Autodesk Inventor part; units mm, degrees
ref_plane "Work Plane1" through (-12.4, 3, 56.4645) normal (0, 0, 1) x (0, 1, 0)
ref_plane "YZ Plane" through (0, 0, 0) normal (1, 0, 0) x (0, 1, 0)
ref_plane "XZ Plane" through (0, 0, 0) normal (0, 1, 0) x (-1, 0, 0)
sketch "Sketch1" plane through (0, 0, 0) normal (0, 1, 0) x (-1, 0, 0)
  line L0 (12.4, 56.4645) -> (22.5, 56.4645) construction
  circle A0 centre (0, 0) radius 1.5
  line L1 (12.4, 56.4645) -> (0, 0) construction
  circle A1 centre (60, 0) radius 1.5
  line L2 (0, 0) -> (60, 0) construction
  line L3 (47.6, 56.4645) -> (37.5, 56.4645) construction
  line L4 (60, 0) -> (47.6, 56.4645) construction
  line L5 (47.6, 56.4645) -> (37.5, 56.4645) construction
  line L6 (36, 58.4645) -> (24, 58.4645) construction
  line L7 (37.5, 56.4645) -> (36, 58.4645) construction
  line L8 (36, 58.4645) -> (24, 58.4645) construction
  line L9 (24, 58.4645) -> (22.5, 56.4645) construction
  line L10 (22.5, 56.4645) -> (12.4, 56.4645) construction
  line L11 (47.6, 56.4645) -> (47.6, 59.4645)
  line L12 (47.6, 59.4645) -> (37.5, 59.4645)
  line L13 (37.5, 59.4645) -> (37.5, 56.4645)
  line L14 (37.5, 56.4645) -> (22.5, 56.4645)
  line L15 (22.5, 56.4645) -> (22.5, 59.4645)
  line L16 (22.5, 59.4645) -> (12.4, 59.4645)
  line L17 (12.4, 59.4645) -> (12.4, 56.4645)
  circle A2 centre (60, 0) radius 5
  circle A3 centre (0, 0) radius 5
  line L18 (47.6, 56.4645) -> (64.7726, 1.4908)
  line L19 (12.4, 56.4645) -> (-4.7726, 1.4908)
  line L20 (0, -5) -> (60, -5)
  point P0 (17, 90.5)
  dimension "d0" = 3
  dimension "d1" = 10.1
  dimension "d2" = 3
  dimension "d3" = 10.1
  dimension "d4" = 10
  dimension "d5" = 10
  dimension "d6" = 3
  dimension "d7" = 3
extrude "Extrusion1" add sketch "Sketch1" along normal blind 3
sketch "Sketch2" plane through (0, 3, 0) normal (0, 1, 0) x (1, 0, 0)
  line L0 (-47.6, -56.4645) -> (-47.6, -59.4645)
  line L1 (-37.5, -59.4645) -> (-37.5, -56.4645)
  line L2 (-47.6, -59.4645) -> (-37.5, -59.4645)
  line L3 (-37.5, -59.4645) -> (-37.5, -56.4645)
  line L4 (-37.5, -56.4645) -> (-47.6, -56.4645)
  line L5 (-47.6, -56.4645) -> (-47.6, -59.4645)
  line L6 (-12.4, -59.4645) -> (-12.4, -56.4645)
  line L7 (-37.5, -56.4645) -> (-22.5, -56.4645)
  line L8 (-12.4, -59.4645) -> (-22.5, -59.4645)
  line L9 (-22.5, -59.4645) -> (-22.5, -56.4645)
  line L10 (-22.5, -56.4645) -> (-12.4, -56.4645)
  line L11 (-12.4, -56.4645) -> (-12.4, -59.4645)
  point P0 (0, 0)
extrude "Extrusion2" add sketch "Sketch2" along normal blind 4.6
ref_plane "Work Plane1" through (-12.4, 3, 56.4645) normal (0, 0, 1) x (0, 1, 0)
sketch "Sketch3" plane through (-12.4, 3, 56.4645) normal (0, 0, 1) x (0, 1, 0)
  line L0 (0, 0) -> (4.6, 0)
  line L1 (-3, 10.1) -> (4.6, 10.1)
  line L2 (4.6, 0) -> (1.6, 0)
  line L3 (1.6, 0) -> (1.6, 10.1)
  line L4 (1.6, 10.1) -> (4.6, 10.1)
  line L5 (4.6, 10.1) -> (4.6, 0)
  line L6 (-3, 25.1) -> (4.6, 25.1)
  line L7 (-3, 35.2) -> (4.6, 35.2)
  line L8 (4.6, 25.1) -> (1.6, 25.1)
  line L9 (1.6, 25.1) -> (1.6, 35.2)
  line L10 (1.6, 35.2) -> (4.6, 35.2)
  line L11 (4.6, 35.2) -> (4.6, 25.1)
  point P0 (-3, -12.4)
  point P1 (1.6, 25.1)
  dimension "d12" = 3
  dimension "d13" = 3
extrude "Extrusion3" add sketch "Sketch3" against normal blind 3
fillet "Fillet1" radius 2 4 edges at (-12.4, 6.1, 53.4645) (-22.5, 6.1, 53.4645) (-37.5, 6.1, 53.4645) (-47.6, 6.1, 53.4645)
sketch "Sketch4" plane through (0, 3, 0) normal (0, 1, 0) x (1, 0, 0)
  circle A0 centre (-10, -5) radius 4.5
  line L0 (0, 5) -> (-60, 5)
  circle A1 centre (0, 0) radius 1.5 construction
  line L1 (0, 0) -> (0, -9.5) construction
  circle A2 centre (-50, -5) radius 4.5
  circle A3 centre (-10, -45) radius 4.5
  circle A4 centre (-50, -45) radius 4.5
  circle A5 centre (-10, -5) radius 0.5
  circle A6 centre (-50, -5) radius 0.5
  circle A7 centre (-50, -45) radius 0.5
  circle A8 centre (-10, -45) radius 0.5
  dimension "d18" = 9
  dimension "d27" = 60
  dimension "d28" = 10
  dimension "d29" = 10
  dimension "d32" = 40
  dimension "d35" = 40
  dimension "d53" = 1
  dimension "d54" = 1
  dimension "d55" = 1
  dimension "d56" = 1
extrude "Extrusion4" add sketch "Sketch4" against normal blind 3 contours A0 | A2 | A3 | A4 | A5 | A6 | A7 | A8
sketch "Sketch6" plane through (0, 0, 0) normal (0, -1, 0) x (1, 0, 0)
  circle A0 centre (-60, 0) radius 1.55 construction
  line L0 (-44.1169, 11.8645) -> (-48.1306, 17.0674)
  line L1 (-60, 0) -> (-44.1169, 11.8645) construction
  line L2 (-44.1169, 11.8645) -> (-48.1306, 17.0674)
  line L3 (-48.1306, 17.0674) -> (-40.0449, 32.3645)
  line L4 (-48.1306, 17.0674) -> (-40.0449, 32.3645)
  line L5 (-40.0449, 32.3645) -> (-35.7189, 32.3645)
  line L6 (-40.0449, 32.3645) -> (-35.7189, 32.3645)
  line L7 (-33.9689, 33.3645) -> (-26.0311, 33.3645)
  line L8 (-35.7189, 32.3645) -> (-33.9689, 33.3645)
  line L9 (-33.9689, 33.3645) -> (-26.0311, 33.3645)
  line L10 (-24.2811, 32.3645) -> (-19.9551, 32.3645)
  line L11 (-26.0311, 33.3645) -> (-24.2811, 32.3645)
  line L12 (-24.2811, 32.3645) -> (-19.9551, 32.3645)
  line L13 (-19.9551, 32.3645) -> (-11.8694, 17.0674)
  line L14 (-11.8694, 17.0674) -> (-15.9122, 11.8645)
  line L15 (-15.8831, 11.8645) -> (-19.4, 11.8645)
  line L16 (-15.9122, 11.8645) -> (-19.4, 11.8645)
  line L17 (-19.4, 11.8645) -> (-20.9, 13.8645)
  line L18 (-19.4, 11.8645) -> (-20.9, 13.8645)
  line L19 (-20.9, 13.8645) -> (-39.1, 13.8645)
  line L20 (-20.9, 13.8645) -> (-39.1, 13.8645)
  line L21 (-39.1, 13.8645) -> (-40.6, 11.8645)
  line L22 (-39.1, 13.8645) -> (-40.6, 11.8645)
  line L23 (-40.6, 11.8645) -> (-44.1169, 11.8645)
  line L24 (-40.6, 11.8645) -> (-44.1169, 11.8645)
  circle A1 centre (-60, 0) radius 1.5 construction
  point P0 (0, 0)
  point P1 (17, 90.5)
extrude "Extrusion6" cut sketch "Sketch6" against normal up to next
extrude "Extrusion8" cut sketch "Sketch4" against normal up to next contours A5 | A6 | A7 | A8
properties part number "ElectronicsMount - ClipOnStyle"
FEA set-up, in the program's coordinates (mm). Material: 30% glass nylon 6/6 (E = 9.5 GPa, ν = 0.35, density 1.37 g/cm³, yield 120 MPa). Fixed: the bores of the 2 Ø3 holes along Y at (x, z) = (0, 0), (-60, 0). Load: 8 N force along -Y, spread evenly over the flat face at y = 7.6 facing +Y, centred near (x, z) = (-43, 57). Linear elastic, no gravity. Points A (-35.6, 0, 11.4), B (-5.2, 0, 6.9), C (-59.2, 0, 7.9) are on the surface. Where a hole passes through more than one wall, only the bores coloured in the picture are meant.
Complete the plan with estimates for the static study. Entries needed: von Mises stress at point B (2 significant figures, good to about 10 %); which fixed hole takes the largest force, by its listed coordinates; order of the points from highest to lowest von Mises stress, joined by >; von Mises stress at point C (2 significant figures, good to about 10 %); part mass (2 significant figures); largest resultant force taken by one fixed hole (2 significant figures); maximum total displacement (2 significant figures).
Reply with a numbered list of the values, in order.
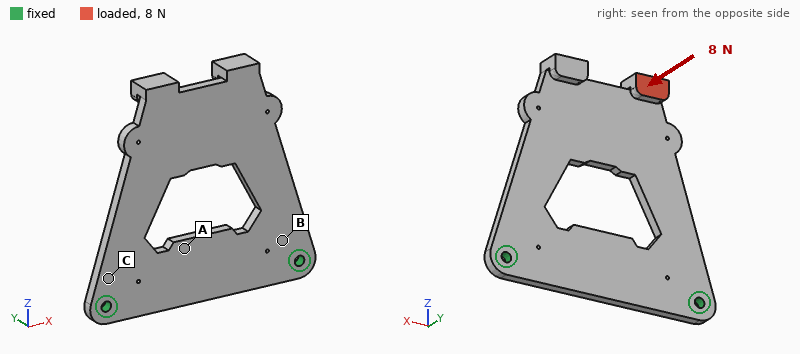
1. 5.9 MPa
2. (-60, 0)
3. C > B > A
4. 9.0 MPa
5. 12 g
6. 5.7 N
7. 0.96 mm
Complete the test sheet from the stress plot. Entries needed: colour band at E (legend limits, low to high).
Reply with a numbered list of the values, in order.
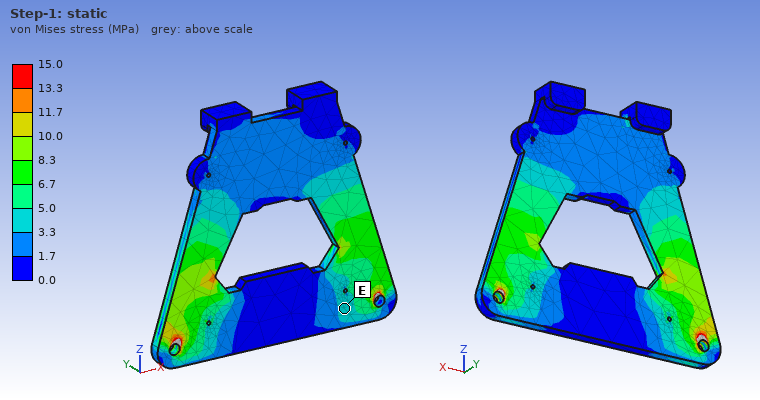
1. 3.3 to 5.0 MPa
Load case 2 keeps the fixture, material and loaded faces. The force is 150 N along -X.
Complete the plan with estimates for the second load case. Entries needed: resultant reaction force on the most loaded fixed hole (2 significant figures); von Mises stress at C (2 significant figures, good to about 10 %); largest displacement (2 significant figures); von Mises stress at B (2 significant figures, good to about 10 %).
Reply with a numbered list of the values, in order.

1. 160 N
2. 16 MPa
3. 0.68 mm
4. 11 MPa
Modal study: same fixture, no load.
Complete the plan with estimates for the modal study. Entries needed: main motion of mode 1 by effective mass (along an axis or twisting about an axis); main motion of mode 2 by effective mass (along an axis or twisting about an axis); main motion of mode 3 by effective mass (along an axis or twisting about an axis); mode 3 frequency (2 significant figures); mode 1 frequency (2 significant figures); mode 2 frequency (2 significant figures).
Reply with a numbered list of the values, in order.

1. along Y
2. twisting about Z
3. along Y
4. 1700 Hz
5. 280 Hz
6. 1000 Hz
